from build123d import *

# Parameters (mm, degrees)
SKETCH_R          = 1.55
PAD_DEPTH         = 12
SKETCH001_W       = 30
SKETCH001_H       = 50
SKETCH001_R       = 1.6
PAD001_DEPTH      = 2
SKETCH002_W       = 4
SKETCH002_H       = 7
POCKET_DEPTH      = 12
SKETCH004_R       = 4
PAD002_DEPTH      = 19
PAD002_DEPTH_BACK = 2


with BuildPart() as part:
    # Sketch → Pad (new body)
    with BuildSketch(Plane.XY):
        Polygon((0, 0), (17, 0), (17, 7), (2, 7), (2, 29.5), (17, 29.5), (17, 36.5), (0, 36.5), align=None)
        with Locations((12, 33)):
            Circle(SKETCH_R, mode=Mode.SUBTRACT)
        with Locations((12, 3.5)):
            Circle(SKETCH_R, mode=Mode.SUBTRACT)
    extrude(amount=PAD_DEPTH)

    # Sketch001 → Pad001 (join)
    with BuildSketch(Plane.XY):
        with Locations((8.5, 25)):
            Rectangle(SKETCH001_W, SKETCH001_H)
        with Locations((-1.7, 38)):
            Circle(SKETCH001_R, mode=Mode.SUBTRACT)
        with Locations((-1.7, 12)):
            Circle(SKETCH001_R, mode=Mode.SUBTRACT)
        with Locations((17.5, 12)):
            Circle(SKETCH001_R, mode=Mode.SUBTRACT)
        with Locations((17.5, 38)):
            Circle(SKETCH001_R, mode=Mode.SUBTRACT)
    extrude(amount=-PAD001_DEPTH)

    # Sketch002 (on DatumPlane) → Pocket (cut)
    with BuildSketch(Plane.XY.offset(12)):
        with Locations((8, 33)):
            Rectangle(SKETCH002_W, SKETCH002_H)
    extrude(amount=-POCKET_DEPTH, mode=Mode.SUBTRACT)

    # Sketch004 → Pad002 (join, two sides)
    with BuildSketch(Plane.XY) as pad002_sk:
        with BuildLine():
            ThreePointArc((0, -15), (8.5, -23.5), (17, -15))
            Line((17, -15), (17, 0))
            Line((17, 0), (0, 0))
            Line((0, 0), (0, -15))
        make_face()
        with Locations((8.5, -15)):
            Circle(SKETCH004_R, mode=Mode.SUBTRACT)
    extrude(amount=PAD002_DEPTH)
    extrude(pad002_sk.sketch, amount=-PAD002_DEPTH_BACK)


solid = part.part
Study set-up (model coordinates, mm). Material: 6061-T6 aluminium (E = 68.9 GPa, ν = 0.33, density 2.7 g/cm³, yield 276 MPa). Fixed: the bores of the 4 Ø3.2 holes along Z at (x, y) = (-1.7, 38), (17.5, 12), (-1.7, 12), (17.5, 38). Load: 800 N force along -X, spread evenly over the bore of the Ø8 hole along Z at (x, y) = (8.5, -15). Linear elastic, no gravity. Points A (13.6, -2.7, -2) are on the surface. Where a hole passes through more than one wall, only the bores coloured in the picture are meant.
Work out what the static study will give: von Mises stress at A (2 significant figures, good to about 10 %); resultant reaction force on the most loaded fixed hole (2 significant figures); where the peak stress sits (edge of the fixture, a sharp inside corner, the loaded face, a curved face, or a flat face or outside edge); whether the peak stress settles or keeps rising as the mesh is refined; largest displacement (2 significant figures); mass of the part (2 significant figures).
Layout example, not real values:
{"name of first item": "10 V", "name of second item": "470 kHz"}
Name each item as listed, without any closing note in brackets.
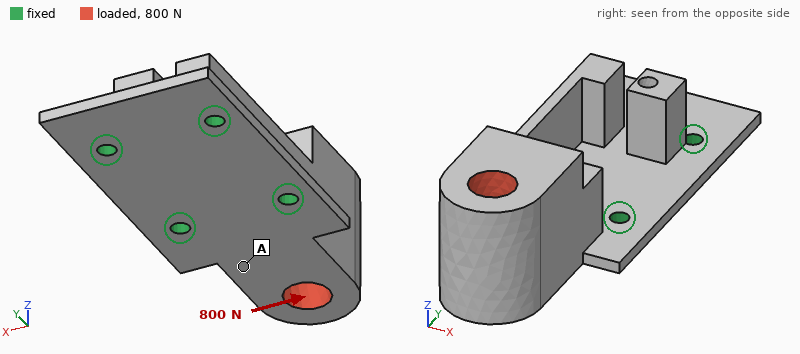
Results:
{"von Mises stress at A": "18 MPa", "resultant reaction force on the most loaded fixed hole": "1.2 kN", "where the peak stress sits": "edge of the fixture", "whether the peak stress settles or keeps rising as the mesh is refined": "keeps rising", "largest displacement": "85 µm", "mass of the part": "34 g"}
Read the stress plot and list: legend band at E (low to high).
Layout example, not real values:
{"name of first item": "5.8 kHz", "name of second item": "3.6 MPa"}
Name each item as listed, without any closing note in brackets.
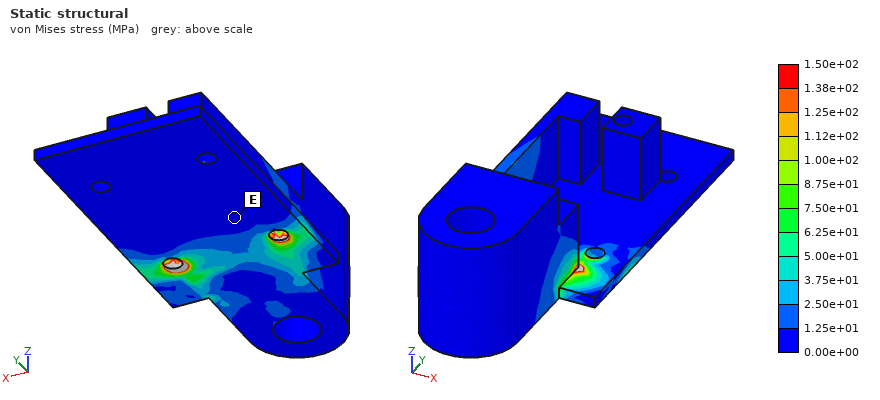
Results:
{"legend band at E": "0.00e+00 to 1.25e+01 MPa"}
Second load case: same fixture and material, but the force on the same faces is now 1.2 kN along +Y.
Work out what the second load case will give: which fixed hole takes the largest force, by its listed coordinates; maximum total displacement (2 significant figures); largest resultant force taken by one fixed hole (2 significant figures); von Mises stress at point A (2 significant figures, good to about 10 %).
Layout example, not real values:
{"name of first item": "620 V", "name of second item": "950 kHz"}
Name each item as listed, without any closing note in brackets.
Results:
{"which fixed hole takes the largest force, by its listed coordinates": "(-1.7, 38)", "maximum total displacement": "0.14 mm", "largest resultant force taken by one fixed hole": "580 N", "von Mises stress at point A": "14 MPa"}
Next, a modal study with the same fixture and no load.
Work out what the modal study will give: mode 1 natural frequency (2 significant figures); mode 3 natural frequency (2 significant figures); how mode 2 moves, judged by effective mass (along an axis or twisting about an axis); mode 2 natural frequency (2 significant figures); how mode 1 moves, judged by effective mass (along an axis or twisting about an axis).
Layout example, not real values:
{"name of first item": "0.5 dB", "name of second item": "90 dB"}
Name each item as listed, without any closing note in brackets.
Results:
{"mode 1 natural frequency": "2500 Hz", "mode 3 natural frequency": "9600 Hz", "how mode 2 moves, judged by effective mass": "along X", "mode 2 natural frequency": "4800 Hz", "how mode 1 moves, judged by effective mass": "along Z"}
